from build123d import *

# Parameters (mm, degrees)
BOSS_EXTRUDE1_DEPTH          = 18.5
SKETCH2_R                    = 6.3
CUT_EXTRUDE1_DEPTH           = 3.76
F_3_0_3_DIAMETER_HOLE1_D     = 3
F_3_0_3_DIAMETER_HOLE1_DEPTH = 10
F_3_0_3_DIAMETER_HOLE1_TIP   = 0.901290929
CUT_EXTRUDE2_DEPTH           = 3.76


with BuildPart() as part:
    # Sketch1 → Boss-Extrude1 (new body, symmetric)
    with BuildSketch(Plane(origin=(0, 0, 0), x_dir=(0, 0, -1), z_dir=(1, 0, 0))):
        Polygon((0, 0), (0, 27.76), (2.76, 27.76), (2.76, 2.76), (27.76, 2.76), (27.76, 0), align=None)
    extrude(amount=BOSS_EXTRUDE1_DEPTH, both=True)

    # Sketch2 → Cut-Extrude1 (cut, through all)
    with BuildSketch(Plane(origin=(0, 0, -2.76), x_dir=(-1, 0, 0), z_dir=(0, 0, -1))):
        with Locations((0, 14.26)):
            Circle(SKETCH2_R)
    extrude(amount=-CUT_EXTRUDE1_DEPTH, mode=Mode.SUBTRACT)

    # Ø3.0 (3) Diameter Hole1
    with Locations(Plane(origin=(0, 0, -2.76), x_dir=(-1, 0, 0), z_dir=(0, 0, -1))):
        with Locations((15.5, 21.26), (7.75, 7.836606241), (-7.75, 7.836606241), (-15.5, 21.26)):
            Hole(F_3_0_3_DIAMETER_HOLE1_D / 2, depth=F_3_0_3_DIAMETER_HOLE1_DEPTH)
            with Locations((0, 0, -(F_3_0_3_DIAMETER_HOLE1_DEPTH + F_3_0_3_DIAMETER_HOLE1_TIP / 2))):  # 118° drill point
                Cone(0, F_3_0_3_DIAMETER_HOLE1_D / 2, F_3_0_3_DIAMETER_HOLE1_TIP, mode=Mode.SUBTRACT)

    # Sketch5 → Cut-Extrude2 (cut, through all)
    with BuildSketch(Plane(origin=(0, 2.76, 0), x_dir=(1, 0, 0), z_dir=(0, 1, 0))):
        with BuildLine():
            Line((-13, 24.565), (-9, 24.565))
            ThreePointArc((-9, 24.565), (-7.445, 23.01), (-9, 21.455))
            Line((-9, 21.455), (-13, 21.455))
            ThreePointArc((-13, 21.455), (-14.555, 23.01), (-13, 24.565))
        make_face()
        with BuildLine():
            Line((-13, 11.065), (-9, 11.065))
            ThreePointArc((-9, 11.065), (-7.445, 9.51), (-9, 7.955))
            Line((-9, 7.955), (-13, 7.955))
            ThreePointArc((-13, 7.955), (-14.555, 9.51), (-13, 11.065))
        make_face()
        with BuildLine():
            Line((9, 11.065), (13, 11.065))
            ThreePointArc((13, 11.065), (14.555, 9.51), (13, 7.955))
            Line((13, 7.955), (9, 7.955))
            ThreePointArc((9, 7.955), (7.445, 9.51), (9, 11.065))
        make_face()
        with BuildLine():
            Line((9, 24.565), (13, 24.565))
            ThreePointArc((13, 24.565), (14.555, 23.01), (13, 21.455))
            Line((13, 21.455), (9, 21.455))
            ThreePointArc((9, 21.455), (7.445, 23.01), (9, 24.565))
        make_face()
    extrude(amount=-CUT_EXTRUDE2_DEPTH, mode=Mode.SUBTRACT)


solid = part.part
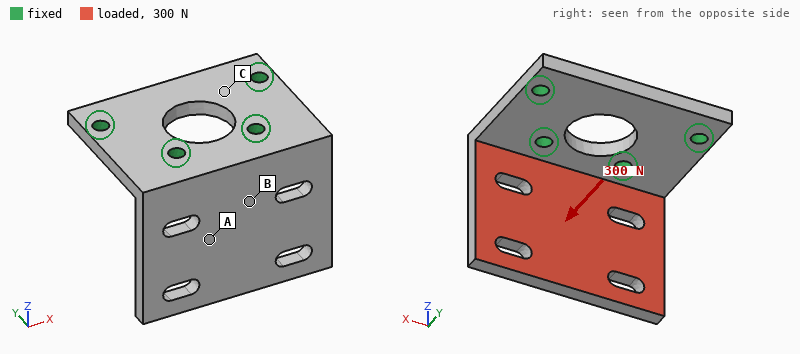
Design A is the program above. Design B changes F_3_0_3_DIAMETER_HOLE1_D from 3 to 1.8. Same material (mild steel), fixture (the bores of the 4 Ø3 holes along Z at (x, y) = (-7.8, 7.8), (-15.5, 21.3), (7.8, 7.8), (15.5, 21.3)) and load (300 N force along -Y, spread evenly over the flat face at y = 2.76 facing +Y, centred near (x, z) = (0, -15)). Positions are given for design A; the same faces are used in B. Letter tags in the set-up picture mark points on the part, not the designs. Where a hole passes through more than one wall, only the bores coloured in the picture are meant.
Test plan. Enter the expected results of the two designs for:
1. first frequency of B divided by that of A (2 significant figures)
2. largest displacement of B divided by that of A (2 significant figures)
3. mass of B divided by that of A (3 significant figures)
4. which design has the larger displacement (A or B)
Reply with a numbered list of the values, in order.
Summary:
1. 0.96
2. 1.1
3. 1.01
4. B
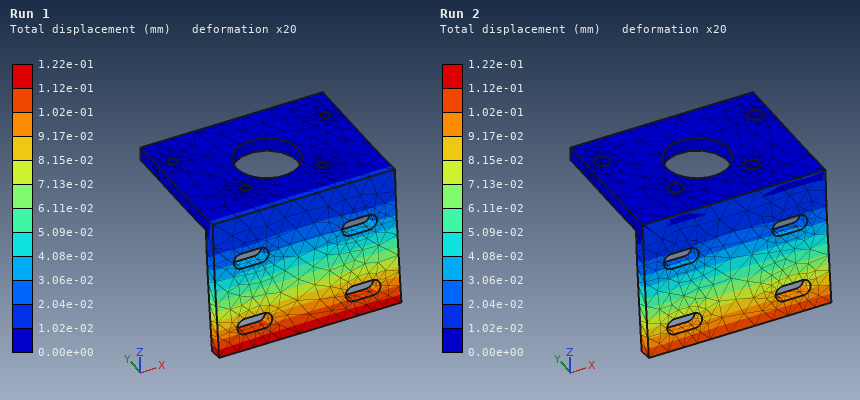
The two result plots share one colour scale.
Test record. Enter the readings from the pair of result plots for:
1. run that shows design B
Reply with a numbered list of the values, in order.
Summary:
1. Run 1
